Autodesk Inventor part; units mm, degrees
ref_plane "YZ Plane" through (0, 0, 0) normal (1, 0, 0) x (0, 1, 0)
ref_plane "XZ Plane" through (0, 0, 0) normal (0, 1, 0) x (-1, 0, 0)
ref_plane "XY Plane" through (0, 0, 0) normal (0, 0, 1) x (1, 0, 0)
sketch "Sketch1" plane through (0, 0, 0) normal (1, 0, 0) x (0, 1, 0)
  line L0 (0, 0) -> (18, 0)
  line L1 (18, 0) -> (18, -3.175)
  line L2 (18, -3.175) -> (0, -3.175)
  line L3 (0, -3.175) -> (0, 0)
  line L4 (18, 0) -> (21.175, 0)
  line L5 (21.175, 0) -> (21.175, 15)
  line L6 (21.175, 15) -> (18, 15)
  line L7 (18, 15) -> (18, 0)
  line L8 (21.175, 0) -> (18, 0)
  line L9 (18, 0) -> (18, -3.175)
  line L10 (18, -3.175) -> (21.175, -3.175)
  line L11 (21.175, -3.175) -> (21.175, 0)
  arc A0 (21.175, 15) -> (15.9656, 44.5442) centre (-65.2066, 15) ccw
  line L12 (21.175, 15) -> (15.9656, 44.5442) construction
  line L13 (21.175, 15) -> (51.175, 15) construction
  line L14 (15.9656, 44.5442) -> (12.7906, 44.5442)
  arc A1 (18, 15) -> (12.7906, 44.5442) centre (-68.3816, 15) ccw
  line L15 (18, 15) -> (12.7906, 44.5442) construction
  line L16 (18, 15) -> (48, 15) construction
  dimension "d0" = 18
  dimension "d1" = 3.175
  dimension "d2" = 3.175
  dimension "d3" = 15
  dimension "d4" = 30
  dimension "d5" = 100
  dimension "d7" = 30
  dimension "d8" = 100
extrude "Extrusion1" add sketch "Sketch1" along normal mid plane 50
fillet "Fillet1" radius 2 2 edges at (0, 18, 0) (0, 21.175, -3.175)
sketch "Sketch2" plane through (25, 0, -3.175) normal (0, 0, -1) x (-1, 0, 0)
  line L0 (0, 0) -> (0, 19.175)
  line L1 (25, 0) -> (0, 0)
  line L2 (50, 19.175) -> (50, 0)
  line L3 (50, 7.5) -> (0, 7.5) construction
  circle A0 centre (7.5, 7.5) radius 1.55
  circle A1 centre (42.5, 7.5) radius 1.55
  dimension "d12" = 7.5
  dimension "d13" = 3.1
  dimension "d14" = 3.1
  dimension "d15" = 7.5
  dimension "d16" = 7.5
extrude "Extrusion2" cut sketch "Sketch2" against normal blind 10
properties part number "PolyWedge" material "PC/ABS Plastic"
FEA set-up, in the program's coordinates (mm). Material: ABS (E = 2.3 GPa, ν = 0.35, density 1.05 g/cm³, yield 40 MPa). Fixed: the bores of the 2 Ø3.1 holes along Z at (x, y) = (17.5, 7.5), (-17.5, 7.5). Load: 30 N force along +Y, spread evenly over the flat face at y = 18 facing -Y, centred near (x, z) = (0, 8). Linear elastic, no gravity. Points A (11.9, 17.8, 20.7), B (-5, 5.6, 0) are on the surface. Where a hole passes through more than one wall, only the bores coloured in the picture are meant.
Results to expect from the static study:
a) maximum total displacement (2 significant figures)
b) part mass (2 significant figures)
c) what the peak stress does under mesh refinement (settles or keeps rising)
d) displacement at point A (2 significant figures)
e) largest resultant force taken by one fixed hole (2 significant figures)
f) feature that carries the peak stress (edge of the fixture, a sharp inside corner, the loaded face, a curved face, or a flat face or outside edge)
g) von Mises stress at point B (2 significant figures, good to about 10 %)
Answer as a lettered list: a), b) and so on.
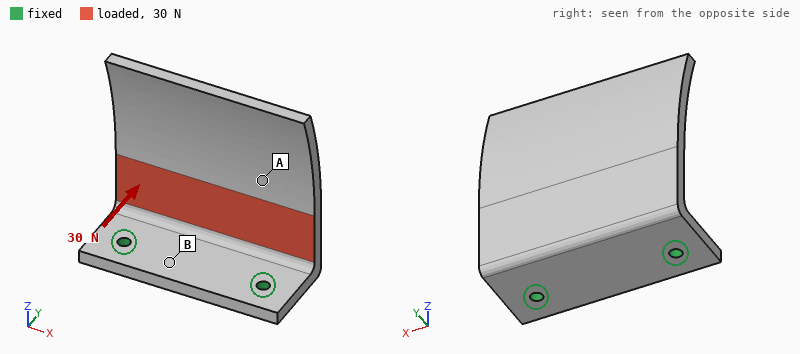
a) 0.71 mm
b) 11 g
c) keeps rising
d) 0.34 mm
e) 15 N
f) edge of the fixture
g) 1.2 MPa
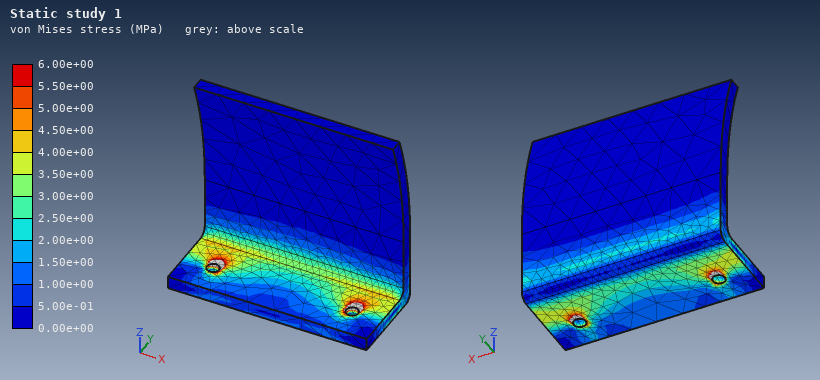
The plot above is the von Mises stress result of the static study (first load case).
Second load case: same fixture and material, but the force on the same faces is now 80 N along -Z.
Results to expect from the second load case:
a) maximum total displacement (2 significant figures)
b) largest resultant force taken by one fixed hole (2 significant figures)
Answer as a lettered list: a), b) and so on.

a) 0.73 mm
b) 40 N
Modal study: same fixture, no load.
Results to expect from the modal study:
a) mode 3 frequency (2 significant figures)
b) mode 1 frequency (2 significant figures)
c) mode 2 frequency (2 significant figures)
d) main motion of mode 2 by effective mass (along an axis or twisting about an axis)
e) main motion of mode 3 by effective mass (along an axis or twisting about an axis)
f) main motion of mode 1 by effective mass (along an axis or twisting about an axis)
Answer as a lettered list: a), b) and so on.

a) 1000 Hz
b) 260 Hz
c) 640 Hz
d) along X
e) along X
f) along Y
